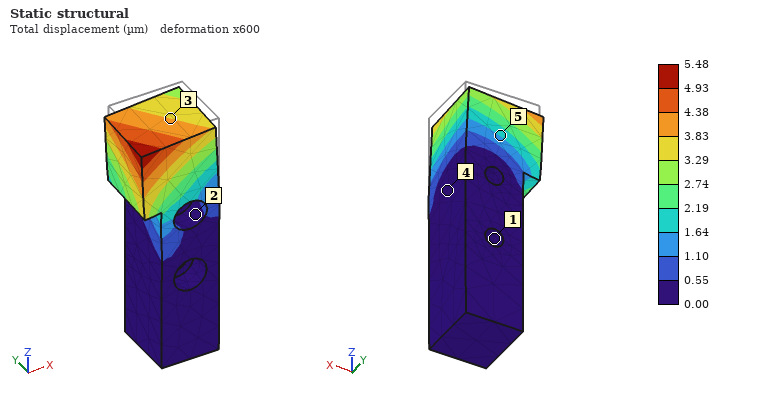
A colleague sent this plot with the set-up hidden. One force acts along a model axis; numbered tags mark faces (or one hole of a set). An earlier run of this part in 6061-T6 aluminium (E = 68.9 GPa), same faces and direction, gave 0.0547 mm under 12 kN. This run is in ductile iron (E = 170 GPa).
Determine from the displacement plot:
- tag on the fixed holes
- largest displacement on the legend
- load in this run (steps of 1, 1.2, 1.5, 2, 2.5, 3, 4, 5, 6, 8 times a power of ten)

1
5.48 µm
3 kN
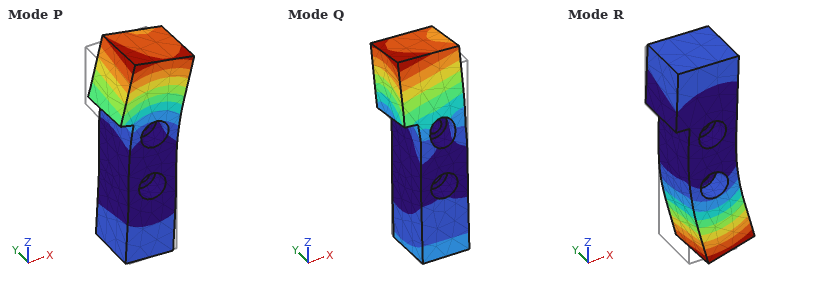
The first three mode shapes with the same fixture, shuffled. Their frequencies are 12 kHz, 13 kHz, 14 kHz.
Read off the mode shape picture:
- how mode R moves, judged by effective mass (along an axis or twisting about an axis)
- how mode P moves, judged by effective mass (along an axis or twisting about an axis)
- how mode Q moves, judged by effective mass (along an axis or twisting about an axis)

along X
along X
along Y
